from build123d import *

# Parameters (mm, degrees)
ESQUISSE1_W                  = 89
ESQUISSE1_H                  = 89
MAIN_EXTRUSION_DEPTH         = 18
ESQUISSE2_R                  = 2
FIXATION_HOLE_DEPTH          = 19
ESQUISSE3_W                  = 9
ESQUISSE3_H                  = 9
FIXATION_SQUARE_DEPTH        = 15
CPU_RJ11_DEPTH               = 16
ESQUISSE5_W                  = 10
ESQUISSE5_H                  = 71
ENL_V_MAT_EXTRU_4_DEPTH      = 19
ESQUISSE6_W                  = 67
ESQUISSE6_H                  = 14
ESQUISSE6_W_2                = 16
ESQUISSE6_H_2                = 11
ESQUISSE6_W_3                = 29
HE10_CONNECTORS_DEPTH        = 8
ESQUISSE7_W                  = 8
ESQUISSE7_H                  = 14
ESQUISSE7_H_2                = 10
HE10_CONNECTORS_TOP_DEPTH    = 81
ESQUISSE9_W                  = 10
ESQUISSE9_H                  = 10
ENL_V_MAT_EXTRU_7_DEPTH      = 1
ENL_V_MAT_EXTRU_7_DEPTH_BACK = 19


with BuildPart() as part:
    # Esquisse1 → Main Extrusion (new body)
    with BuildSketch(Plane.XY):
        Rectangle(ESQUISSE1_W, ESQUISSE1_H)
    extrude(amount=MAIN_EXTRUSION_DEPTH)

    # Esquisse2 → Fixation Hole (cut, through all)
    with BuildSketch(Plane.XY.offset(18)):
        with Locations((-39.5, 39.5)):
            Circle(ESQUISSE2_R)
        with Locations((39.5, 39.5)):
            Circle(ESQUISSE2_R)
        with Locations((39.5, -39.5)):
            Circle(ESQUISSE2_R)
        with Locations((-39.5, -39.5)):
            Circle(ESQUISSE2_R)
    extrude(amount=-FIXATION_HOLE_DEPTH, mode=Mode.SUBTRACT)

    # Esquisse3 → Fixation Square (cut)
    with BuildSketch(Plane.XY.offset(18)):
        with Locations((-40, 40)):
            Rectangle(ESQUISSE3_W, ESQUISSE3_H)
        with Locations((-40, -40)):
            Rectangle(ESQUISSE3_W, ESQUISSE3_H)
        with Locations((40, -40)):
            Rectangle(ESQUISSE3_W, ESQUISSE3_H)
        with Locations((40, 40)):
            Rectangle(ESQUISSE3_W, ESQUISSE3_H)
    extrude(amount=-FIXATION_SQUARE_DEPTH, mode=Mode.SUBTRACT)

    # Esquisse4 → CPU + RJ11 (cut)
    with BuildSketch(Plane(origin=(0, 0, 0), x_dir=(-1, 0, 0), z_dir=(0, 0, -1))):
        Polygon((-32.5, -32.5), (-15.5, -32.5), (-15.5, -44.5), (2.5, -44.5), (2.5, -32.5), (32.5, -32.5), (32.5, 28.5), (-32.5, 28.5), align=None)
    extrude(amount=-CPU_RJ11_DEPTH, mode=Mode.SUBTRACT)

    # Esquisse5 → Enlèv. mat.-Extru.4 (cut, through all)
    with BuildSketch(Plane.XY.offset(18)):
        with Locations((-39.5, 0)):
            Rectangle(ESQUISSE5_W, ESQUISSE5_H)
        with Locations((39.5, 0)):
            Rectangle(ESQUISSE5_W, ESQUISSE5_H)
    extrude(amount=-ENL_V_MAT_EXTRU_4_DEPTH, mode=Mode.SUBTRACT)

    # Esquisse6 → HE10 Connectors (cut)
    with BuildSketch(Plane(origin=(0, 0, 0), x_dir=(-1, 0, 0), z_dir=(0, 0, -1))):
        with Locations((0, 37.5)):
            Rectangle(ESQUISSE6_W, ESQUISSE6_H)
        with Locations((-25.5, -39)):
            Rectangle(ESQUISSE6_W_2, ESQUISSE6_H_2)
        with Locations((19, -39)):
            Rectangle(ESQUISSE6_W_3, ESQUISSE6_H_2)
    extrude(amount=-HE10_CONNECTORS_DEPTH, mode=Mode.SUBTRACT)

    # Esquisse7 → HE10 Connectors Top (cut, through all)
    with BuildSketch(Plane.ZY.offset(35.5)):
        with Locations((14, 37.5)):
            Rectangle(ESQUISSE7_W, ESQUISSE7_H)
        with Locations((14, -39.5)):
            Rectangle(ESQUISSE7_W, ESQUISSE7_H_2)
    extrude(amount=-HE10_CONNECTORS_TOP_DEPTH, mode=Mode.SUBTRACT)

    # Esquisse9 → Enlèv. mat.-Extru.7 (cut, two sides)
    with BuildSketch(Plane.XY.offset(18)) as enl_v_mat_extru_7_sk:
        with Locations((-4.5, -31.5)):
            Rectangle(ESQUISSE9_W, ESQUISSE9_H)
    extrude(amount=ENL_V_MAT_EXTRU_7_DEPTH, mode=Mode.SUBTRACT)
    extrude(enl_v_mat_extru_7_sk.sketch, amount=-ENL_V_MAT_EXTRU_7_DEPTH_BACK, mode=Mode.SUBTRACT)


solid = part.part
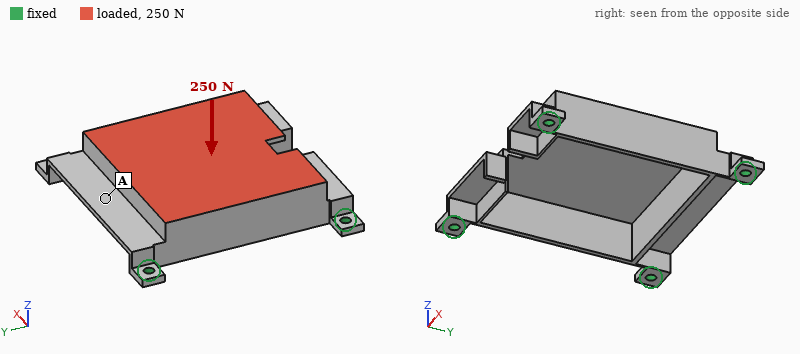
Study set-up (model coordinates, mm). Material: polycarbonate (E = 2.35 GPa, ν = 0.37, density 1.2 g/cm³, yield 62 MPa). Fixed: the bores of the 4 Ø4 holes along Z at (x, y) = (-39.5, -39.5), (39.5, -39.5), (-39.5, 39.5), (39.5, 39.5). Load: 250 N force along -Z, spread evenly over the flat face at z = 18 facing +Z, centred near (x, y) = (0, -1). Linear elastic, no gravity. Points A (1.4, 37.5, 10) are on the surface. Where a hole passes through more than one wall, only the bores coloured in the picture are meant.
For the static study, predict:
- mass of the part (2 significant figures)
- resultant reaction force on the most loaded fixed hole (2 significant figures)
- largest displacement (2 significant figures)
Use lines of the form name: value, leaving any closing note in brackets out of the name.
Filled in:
mass of the part: 25 g
resultant reaction force on the most loaded fixed hole: 110 N
largest displacement: 1.4 mm
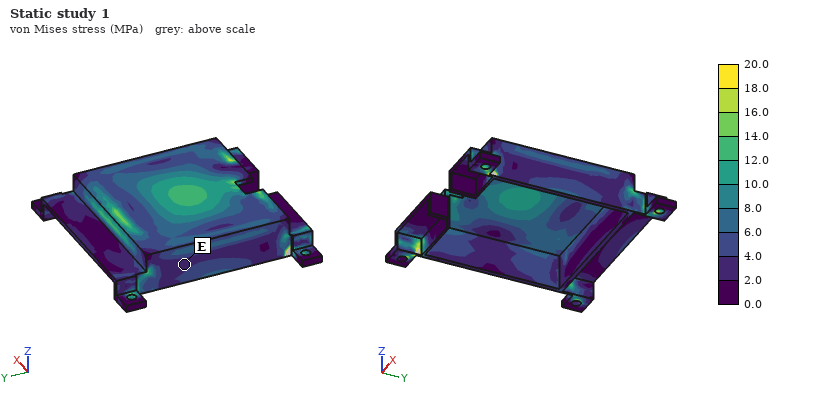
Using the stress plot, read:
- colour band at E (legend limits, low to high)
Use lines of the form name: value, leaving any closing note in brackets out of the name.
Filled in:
colour band at E: 2.0 to 4.0 MPa
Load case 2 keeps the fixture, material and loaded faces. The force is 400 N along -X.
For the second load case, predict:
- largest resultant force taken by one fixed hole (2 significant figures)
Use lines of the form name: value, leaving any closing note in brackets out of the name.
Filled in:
largest resultant force taken by one fixed hole: 190 N
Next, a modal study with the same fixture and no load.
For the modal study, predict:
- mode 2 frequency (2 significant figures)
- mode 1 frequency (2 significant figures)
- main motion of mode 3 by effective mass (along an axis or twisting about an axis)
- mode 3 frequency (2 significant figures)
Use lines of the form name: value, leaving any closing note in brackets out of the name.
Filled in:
mode 2 frequency: 780 Hz
mode 1 frequency: 750 Hz
main motion of mode 3 by effective mass: along X
mode 3 frequency: 910 Hz
